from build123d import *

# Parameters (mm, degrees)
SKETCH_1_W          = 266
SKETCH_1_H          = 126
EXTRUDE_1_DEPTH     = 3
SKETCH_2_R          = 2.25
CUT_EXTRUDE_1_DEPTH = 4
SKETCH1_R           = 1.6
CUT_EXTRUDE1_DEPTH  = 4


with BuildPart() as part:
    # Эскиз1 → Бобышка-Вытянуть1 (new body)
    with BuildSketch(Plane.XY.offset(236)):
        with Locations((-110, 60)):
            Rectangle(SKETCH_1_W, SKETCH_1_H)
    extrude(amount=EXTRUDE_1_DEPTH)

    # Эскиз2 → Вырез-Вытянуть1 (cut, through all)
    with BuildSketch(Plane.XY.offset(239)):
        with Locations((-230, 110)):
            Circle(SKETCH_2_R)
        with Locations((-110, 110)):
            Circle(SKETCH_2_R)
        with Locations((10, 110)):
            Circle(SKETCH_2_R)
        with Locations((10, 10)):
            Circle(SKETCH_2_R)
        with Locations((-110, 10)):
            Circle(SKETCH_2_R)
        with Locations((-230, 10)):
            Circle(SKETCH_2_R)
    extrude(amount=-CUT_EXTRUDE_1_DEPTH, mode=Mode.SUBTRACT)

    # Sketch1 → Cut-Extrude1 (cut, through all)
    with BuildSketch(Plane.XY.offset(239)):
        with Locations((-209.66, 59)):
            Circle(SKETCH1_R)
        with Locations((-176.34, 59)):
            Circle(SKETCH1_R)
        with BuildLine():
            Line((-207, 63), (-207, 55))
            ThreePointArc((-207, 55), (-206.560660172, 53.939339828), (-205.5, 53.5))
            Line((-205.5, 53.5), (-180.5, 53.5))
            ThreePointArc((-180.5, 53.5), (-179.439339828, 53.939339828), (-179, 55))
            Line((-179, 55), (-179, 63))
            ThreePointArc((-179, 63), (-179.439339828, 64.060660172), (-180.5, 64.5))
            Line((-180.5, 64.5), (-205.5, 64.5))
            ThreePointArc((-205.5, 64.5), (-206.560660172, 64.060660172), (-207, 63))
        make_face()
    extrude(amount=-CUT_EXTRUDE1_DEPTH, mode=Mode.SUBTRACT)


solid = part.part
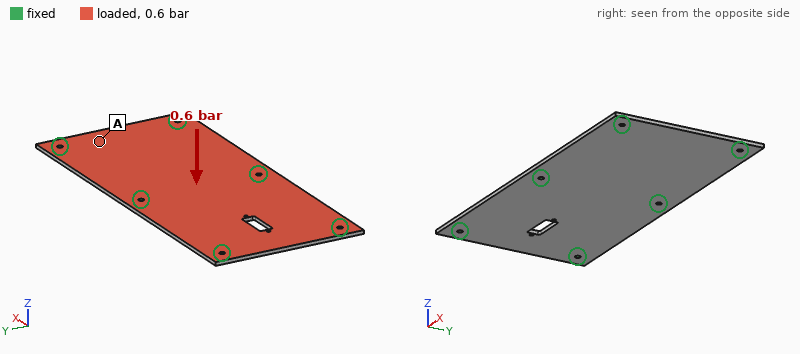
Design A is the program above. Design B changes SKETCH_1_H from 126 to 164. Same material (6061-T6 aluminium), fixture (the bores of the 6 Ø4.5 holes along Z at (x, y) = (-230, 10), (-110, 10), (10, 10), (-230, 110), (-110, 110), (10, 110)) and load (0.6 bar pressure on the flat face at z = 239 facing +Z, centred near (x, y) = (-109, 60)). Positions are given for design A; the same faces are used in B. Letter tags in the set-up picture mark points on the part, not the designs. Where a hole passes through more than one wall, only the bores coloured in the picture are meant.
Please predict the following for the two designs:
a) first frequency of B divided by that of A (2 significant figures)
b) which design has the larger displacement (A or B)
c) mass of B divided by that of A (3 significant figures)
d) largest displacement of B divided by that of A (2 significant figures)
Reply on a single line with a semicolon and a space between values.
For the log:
0.99; A; 1.31; 0.91
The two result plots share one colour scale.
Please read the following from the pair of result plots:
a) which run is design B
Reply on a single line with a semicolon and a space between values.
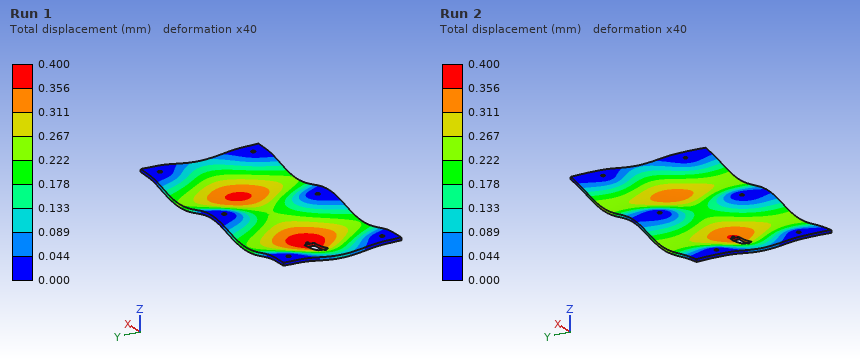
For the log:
Run 2
